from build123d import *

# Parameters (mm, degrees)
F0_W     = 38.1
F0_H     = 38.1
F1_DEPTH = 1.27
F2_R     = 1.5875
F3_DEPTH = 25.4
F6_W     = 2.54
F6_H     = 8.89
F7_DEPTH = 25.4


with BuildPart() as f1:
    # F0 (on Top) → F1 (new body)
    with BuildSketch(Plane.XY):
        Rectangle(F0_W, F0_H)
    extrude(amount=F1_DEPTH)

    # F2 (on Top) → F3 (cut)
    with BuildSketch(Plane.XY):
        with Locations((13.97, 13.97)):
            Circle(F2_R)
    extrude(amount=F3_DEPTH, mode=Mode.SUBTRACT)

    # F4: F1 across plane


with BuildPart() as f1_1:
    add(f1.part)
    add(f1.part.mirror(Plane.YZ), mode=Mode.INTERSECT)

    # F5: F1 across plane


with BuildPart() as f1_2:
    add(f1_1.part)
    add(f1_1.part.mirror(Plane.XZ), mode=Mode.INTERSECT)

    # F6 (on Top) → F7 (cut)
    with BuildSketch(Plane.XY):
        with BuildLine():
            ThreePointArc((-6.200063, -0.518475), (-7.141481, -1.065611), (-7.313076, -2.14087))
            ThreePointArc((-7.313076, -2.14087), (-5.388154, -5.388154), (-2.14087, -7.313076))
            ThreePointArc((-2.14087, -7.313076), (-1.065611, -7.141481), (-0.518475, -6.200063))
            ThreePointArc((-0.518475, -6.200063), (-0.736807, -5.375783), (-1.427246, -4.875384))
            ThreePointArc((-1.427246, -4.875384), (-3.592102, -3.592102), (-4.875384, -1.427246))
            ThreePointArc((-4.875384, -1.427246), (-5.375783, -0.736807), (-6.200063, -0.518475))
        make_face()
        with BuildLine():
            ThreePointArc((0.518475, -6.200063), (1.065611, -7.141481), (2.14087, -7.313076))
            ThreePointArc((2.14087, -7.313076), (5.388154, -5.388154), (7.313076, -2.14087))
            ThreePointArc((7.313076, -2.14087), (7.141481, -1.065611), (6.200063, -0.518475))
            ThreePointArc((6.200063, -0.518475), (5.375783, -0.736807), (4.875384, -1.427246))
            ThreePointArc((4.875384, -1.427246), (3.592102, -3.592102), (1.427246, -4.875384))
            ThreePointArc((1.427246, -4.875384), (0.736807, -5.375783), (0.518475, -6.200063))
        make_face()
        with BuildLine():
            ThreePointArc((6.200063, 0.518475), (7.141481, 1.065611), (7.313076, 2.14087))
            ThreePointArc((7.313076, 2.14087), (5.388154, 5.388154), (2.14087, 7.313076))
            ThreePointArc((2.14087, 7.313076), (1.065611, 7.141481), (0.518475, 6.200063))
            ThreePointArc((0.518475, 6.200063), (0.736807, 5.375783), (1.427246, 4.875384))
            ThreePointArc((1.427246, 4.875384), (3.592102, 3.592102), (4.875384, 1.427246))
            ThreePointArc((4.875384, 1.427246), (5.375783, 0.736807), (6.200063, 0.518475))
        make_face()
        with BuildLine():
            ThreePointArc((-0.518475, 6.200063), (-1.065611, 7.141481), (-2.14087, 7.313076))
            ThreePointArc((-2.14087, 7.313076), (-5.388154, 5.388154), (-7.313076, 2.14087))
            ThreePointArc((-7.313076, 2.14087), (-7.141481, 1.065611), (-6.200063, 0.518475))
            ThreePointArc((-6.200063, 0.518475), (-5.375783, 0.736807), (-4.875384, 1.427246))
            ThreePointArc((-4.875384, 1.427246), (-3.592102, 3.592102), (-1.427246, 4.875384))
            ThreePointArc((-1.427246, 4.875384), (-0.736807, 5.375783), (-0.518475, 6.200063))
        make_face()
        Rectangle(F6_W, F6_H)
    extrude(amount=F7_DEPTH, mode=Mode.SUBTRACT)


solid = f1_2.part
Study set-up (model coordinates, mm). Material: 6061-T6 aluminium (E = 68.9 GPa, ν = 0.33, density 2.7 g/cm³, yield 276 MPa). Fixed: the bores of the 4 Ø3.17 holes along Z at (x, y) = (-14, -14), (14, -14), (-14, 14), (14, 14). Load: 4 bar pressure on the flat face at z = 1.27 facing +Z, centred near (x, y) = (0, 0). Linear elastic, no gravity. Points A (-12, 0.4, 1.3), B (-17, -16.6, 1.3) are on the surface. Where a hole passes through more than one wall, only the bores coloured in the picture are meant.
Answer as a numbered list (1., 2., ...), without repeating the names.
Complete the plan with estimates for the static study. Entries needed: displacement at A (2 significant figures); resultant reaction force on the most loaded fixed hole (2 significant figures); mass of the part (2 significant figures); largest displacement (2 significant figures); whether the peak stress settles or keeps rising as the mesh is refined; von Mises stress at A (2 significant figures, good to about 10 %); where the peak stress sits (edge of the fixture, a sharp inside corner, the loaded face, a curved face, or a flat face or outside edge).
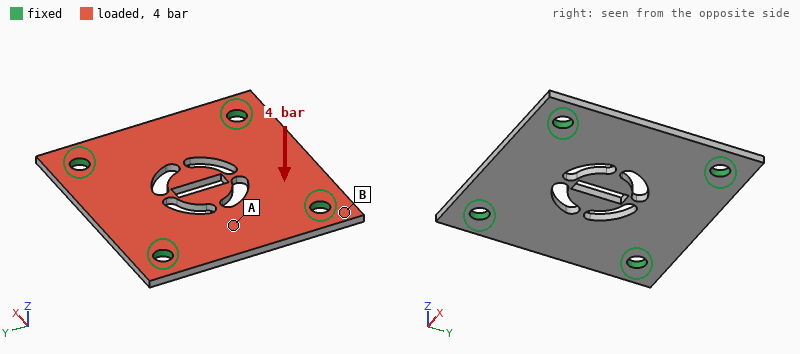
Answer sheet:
1. 0.060 mm
2. 130 N
3. 4.5 g
4. 0.11 mm
5. keeps rising
6. 51 MPa
7. edge of the fixture
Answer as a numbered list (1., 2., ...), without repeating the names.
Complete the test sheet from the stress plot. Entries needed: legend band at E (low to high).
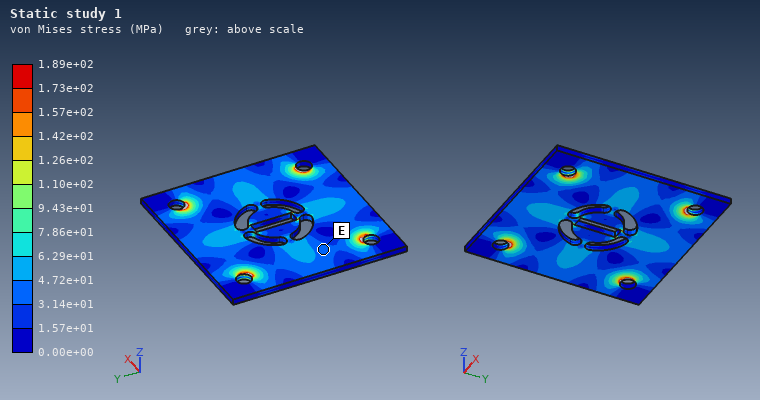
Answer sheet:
1. 3.14e+01 to 4.72e+01 MPa
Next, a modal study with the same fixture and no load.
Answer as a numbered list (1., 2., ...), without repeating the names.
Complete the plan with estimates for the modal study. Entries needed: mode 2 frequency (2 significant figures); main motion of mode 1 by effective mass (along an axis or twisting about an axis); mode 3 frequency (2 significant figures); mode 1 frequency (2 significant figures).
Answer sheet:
1. 9900 Hz
2. along Z
3. 9900 Hz
4. 6700 Hz
